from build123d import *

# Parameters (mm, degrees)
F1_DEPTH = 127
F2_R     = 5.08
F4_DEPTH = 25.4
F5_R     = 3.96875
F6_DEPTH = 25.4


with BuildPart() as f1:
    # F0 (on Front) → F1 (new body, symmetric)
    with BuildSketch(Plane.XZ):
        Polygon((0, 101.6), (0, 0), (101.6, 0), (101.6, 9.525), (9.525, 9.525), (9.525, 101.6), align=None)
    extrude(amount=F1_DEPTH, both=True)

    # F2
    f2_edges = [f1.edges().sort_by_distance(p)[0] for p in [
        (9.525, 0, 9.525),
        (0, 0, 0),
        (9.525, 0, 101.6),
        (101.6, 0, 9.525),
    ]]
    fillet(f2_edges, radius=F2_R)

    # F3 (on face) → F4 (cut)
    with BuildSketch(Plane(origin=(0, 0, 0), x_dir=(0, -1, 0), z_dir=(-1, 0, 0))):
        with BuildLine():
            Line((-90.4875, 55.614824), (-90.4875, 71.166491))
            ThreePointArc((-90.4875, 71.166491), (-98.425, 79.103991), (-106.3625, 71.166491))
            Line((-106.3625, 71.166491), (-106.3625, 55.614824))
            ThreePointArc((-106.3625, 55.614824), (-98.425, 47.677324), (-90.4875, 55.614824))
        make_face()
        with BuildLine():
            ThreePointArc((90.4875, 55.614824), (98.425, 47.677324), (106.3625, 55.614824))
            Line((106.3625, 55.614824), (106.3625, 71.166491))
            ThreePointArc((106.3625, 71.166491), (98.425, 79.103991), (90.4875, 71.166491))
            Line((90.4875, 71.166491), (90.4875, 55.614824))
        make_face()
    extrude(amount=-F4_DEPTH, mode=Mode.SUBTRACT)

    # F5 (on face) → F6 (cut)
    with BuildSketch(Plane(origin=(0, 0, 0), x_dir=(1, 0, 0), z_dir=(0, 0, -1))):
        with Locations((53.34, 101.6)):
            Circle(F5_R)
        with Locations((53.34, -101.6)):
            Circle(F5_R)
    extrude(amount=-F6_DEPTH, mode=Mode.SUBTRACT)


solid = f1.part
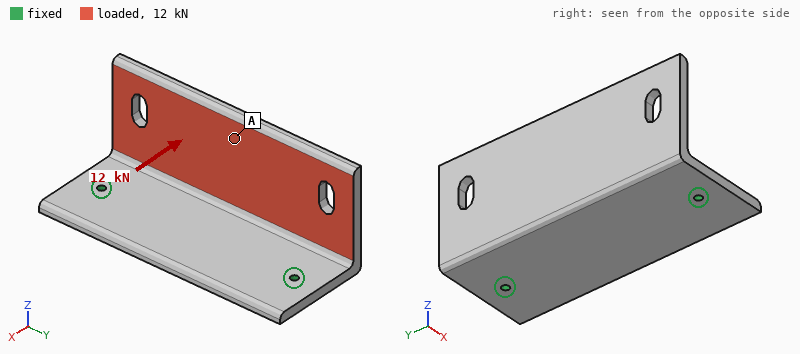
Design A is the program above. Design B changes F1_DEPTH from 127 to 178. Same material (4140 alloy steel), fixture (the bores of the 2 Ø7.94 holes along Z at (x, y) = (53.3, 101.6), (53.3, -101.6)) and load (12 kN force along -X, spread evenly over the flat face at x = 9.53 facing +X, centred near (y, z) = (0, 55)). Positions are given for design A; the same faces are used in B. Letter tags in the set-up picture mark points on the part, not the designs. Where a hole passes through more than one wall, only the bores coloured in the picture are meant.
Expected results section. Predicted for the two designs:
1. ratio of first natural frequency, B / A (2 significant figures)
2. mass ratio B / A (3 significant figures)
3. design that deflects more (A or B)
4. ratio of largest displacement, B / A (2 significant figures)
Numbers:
0.94
1.41
A
0.77
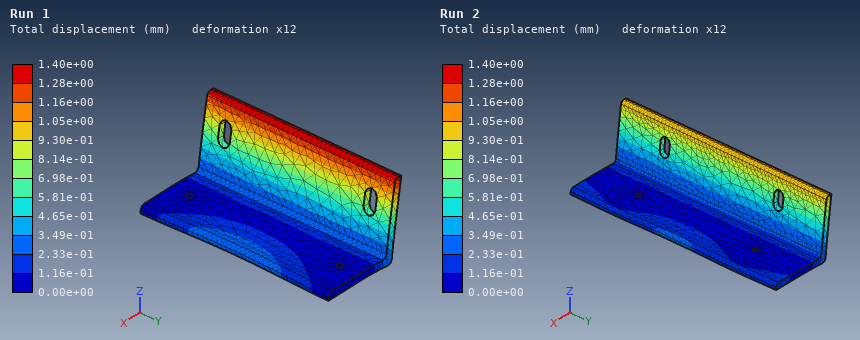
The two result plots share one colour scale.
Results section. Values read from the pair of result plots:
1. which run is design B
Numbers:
Run 2
